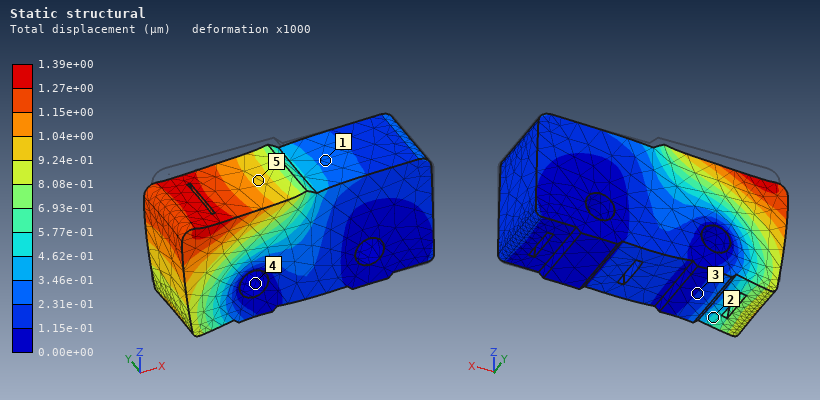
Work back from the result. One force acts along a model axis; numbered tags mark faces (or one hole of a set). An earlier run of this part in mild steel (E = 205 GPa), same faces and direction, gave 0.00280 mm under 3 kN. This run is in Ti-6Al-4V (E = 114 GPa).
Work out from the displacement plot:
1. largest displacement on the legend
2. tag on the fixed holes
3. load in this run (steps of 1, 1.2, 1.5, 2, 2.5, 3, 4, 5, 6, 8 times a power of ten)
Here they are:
1.39e+00 µm
4
800 N
